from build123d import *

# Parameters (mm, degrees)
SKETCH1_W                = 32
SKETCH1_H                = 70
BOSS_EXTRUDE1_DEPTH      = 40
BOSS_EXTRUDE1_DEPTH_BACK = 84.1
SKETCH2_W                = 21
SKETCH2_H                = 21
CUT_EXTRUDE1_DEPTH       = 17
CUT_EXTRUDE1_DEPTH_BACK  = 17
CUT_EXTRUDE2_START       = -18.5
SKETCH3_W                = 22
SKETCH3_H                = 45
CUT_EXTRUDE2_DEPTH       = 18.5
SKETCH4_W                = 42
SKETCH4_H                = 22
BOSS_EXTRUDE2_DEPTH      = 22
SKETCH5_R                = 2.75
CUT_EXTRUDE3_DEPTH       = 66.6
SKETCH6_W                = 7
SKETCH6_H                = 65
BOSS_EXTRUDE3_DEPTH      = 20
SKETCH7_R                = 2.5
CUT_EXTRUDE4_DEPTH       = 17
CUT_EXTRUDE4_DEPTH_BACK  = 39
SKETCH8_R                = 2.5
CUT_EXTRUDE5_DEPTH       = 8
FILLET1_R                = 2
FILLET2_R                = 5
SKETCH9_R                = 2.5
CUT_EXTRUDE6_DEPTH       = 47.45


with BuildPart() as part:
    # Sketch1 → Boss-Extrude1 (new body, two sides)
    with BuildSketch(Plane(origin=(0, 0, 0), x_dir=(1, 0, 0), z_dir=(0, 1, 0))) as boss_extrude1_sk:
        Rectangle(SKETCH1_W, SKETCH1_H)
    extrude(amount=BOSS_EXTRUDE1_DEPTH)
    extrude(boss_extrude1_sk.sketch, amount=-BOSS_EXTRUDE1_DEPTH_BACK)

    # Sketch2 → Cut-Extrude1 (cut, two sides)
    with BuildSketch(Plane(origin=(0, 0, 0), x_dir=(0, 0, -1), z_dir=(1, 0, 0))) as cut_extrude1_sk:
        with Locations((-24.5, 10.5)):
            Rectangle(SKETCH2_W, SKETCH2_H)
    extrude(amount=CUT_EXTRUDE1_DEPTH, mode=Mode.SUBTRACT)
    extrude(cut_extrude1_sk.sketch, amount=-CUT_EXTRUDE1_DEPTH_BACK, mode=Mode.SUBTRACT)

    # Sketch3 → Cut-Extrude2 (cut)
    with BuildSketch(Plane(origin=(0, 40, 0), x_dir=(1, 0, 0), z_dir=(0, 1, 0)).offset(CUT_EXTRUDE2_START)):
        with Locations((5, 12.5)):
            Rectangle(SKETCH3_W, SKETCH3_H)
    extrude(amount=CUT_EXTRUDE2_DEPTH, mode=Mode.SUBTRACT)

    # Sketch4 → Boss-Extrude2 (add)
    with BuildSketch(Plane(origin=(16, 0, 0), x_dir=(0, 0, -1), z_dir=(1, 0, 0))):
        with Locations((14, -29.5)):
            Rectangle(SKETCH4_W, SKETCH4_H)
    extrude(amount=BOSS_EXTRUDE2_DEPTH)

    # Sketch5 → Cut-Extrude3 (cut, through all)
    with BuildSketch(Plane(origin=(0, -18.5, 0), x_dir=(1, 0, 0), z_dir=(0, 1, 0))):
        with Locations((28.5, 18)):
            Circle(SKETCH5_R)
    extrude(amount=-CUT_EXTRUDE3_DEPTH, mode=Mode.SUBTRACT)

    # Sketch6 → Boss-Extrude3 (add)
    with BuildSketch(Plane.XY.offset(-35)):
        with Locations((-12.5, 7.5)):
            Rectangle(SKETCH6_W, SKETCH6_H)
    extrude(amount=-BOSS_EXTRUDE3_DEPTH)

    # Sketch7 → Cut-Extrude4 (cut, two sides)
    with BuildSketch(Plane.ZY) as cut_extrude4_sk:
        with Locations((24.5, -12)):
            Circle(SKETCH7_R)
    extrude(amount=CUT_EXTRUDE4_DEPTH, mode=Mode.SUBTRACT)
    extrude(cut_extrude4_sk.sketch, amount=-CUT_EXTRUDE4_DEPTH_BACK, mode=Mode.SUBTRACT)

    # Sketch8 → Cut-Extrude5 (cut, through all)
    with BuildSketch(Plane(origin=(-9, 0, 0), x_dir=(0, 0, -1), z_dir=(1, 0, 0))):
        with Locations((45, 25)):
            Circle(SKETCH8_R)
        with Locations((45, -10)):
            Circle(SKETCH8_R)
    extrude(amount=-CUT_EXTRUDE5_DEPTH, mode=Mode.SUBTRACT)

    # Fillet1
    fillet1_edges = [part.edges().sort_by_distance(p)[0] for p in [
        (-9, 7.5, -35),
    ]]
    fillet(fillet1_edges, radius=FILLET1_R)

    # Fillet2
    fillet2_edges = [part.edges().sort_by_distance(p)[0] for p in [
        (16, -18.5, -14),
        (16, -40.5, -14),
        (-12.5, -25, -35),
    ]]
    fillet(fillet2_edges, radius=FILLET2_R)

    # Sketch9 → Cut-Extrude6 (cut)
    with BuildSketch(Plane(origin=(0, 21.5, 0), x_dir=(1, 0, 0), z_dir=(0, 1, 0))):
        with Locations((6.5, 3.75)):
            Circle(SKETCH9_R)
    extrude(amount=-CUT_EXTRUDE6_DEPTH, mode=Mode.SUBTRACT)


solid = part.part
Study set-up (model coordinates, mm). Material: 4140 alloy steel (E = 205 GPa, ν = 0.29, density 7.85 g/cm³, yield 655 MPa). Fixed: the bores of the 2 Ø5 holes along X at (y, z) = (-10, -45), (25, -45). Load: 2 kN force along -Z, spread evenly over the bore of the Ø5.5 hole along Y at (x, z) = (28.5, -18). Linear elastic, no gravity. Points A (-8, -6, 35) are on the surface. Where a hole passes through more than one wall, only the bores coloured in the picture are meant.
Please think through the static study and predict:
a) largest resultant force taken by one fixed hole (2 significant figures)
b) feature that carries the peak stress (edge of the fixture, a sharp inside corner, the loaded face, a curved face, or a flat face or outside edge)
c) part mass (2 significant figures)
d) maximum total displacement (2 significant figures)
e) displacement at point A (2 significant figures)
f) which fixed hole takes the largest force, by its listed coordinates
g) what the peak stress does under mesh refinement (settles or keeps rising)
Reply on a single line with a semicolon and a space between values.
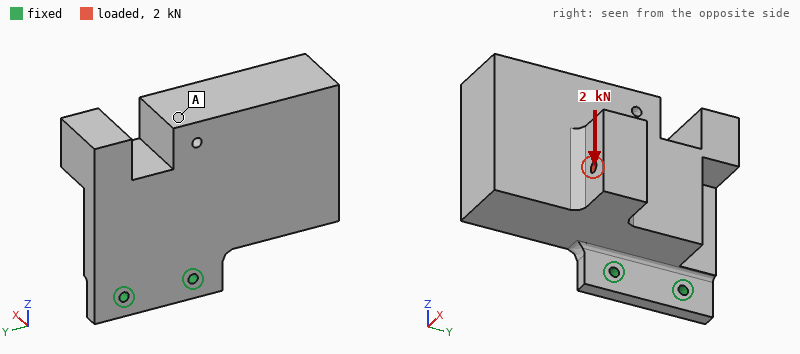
3.0 kN; edge of the fixture; 2.1 kg; 0.27 mm; 0.24 mm; (-10, -45); keeps rising
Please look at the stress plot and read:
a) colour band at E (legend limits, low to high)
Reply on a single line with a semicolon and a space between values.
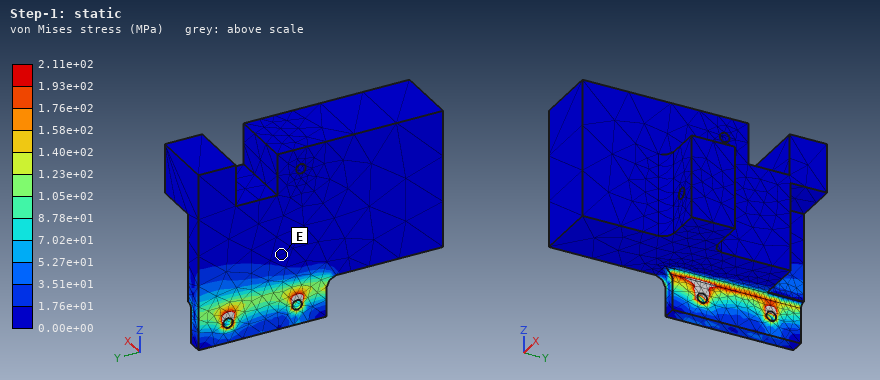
0.00e+00 to 1.76e+01 MPa
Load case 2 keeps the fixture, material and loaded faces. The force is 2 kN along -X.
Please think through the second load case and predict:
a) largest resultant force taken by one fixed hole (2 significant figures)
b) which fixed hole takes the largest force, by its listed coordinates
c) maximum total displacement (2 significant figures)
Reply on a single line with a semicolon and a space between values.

2.8 kN; (-10, -45); 0.18 mm
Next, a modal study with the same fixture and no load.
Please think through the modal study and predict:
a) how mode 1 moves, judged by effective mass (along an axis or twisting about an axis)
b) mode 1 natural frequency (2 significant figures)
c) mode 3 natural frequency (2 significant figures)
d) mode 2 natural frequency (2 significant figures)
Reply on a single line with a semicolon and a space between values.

along X; 360 Hz; 1500 Hz; 1100 Hz
